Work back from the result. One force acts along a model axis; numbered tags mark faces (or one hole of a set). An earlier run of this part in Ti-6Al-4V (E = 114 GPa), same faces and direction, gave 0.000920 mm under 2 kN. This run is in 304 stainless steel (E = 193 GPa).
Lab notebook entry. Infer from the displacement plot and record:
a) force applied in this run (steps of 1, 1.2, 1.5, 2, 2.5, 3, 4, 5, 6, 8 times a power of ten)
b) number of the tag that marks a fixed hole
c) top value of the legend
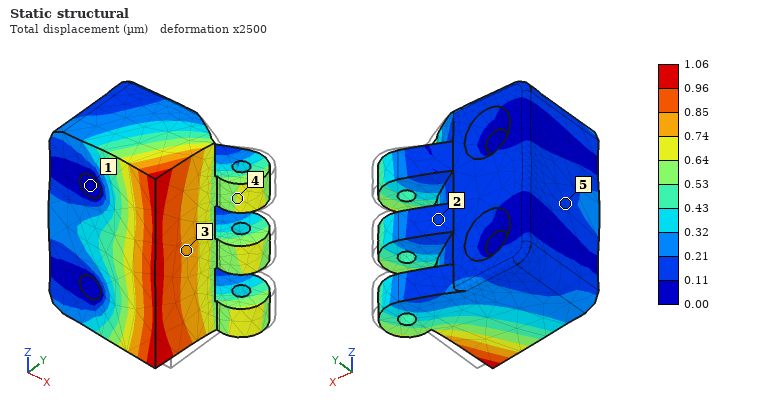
4 kN
1
1.06 µm
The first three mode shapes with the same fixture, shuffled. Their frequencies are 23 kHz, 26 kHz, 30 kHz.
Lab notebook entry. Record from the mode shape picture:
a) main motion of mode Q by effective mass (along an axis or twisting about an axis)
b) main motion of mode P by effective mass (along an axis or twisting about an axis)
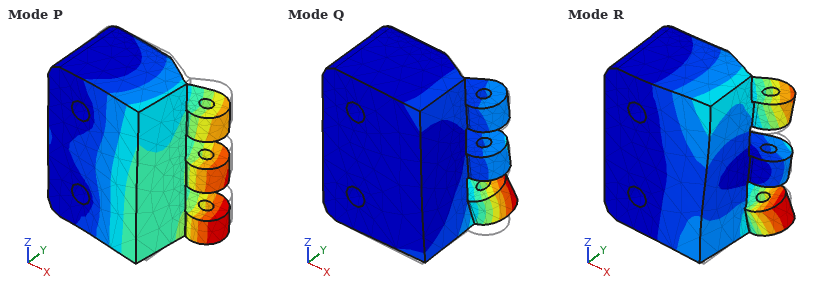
along Z
along Y
